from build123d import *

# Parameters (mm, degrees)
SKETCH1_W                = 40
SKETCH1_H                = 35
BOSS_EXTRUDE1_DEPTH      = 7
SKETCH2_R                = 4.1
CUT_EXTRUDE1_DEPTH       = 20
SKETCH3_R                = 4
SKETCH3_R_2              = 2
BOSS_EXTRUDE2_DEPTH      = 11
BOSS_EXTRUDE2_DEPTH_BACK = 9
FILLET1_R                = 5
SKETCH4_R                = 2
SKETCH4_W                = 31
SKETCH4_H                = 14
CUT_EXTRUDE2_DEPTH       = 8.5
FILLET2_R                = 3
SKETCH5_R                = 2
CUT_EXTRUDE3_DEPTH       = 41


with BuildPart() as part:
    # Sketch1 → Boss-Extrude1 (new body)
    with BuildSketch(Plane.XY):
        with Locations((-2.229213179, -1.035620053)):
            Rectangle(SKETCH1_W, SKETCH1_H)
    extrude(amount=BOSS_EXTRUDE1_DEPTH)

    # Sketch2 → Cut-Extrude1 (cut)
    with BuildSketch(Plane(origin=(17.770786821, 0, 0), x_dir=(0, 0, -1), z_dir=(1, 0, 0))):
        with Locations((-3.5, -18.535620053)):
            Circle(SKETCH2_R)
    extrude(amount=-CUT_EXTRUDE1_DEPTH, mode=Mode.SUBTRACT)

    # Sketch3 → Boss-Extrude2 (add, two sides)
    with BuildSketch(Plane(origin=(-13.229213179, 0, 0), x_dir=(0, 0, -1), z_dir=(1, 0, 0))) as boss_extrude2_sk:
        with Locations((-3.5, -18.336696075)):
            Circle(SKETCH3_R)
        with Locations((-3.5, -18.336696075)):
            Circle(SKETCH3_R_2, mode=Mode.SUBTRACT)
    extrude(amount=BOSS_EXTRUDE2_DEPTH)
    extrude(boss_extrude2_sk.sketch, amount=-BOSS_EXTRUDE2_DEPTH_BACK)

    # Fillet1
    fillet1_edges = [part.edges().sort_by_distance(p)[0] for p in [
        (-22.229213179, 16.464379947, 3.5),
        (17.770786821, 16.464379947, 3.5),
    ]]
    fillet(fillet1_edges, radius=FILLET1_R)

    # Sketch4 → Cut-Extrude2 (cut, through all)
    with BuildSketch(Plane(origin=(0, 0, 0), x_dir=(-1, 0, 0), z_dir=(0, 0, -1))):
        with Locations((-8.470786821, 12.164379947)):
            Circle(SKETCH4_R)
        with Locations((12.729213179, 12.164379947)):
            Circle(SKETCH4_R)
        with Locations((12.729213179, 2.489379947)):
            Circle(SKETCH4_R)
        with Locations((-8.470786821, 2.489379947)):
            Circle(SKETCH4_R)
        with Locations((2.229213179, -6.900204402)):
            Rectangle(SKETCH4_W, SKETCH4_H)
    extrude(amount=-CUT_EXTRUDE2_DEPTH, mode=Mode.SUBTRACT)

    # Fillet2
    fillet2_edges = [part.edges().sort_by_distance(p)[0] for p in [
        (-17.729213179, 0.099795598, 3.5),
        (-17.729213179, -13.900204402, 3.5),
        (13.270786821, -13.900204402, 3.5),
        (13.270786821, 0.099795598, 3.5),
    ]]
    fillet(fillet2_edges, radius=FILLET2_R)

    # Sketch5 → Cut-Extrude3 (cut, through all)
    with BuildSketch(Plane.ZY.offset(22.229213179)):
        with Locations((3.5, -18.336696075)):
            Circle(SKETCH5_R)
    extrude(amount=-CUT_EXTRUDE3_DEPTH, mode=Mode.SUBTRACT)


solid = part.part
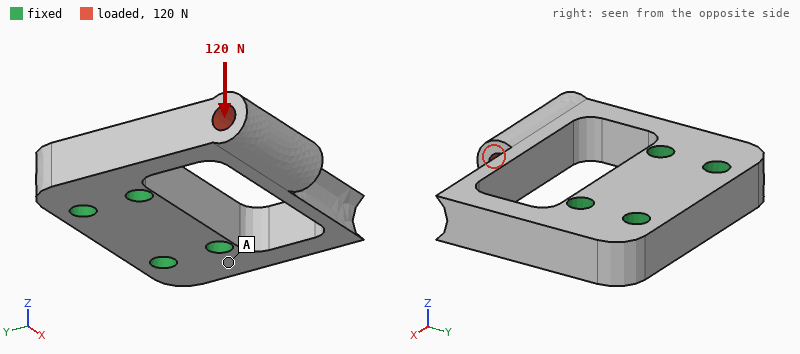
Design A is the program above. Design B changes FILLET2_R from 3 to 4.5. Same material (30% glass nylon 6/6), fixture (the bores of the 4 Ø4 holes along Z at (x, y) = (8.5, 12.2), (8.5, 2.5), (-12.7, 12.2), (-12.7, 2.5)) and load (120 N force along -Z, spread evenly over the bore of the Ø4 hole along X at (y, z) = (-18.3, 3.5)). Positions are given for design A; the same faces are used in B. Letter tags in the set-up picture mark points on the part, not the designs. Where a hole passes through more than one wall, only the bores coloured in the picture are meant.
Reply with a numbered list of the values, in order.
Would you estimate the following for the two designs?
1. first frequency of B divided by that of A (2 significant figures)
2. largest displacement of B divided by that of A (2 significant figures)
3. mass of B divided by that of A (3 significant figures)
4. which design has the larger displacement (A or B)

1. 1.0
2. 0.92
3. 1.01
4. A
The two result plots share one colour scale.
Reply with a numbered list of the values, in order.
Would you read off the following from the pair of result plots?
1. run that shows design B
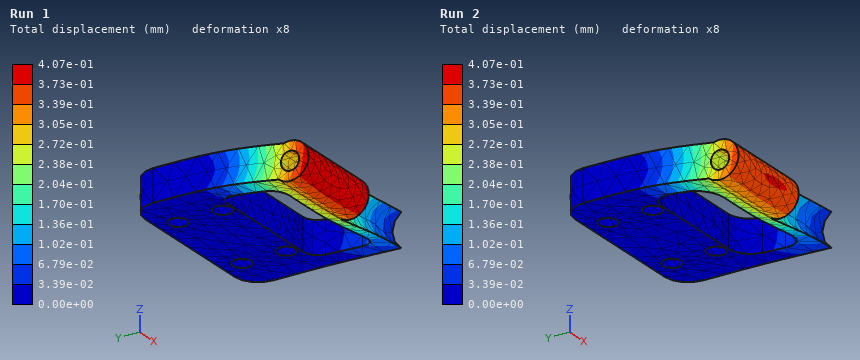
1. Run 2
